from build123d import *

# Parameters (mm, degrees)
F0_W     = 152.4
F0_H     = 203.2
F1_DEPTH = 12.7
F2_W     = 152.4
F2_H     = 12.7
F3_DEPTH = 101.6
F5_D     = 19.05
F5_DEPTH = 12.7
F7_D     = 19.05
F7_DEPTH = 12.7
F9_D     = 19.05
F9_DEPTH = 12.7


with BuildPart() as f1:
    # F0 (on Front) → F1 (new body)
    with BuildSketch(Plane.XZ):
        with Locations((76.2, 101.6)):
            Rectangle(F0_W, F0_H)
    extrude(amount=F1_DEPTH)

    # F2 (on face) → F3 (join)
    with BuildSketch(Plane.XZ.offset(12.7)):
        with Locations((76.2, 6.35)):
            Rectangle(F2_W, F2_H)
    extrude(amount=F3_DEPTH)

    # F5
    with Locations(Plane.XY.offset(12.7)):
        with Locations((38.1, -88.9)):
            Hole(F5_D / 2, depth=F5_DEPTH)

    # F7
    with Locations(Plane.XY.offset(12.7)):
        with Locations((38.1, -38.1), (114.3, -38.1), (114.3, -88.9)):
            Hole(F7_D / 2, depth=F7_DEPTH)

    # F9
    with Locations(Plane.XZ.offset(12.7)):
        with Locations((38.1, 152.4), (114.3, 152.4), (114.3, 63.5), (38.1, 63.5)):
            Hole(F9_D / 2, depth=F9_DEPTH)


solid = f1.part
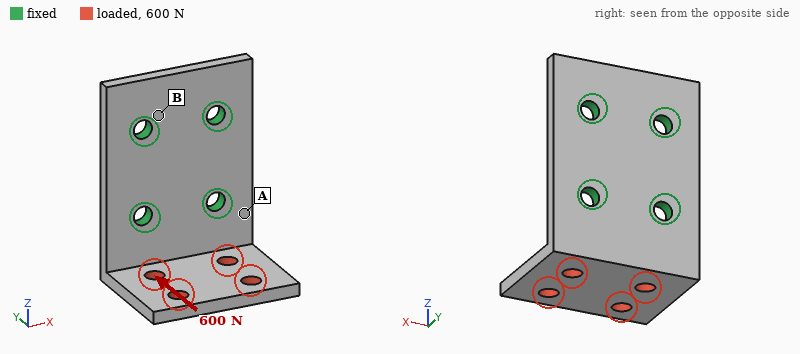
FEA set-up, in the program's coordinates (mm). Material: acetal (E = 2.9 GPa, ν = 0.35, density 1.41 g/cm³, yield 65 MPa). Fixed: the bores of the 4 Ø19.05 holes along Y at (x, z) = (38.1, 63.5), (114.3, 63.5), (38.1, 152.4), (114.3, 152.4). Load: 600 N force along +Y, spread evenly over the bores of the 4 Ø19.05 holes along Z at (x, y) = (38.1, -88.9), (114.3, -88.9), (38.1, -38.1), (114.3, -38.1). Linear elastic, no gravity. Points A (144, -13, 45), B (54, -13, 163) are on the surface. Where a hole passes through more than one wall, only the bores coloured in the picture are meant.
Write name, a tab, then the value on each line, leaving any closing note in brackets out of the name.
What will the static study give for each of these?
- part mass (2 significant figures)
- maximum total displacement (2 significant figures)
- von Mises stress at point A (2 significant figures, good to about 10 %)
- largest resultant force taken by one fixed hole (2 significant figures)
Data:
part mass	790 g
maximum total displacement	1.3 mm
von Mises stress at point A	4.1 MPa
largest resultant force taken by one fixed hole	320 N
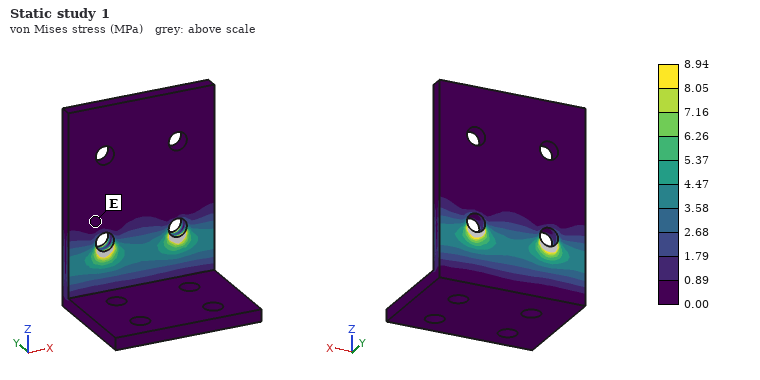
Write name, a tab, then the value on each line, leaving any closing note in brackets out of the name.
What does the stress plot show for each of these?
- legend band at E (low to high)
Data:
legend band at E	0.00 to 0.89 MPa
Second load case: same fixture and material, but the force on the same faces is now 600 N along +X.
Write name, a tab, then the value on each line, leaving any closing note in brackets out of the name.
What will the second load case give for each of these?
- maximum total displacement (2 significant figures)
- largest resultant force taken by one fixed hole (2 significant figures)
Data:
maximum total displacement	0.82 mm
largest resultant force taken by one fixed hole	560 N
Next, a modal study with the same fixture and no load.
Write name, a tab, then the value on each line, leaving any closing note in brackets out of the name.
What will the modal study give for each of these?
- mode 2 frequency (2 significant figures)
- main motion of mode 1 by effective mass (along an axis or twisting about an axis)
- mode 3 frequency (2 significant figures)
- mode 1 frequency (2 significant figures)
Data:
mode 2 frequency	280 Hz
main motion of mode 1 by effective mass	along Z
mode 3 frequency	450 Hz
mode 1 frequency	150 Hz
